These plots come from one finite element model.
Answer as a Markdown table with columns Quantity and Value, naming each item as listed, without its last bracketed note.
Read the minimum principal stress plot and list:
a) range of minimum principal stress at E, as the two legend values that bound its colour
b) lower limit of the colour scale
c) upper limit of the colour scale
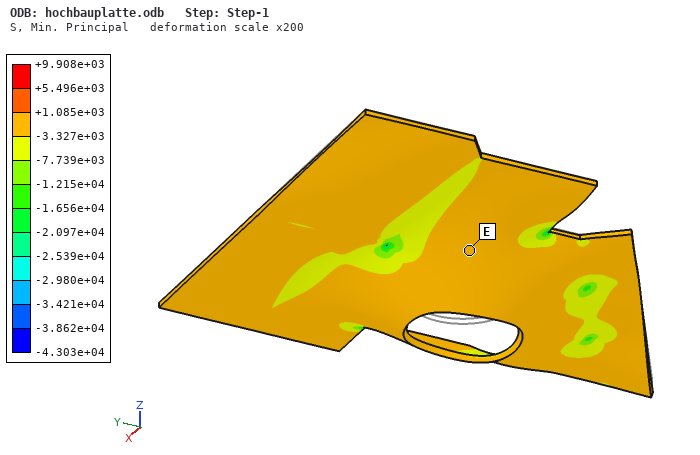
| Quantity | Value |
|---|---|
| range of minimum principal stress at E, as the two legend values that bound its colour | -3.327e+03 to +1.085e+03 |
| lower limit of the colour scale | -4.303e+04 |
| upper limit of the colour scale | +9.908e+03 |
